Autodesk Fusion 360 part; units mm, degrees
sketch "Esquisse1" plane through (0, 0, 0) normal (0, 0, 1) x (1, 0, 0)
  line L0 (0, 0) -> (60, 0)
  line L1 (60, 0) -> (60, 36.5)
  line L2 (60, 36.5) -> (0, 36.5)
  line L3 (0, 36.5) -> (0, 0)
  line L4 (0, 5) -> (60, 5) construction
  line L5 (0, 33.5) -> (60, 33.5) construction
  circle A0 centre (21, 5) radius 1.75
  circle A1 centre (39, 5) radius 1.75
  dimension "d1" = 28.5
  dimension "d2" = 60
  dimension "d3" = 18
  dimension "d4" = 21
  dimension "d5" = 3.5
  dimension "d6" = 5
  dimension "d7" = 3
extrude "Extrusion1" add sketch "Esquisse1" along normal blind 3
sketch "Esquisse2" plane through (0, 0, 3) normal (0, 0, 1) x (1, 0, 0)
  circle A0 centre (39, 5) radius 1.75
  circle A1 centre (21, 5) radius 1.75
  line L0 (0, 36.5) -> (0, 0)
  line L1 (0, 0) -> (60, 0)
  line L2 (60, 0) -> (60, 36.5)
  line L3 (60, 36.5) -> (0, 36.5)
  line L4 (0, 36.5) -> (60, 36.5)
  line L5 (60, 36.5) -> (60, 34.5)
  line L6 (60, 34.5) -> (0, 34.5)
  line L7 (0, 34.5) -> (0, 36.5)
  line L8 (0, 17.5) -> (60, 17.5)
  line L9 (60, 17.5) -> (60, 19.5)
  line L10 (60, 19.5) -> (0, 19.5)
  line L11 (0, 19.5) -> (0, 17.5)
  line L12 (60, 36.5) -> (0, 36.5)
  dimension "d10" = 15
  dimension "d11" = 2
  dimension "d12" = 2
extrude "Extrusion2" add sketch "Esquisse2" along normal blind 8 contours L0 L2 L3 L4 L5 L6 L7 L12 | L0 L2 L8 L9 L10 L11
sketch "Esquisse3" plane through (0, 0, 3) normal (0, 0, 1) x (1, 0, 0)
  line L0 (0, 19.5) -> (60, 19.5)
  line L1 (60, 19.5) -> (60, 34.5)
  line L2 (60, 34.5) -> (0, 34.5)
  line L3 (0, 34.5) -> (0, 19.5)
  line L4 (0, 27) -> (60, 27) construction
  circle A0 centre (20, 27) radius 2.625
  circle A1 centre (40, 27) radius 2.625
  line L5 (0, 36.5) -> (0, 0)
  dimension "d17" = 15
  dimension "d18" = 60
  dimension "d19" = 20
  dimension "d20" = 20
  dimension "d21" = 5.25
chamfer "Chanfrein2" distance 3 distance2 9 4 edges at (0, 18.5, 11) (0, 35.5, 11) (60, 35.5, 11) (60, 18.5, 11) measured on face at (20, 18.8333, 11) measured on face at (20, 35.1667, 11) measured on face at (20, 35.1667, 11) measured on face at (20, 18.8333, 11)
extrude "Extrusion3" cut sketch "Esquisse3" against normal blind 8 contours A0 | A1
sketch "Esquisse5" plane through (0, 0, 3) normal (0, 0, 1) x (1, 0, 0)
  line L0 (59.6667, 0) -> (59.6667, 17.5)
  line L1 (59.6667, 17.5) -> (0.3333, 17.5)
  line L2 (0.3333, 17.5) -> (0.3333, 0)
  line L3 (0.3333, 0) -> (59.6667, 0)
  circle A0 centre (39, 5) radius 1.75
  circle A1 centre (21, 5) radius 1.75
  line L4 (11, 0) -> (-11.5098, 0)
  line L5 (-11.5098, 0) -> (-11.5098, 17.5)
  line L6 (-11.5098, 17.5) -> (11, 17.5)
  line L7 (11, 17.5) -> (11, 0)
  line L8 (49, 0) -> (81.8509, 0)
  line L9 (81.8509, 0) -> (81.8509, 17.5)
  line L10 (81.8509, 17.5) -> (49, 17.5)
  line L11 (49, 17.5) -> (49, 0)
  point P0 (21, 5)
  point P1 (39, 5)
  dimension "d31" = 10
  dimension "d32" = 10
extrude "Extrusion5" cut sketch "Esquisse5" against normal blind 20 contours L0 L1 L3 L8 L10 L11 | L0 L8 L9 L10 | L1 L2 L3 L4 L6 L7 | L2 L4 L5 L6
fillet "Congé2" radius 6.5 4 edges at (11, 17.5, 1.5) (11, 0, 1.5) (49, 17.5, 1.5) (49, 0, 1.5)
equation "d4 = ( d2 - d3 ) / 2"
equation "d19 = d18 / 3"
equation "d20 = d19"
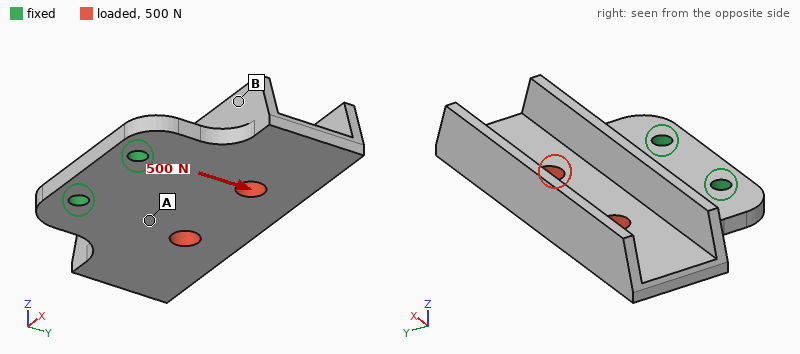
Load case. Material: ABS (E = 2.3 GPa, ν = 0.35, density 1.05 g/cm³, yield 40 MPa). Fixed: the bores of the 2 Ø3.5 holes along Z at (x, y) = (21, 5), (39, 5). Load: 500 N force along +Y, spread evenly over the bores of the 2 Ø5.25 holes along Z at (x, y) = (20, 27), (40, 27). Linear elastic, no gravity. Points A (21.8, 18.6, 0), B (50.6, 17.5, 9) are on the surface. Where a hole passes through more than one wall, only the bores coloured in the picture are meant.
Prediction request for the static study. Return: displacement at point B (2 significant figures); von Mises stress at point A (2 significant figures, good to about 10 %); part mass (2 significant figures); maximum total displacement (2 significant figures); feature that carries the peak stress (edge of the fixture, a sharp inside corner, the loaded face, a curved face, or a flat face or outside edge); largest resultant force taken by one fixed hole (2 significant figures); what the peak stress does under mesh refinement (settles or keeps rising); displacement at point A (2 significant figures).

36 µm
5.7 MPa
7.4 g
70 µm
edge of the fixture
250 N
keeps rising
37 µm
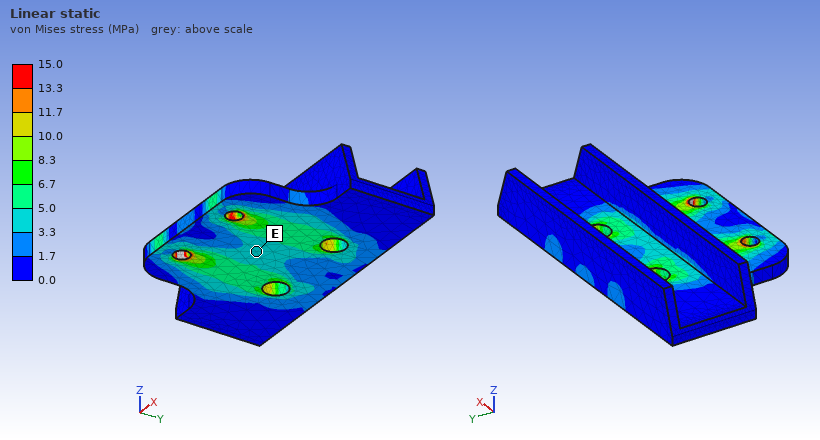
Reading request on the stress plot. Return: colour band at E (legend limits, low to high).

3.3 to 5.0 MPa
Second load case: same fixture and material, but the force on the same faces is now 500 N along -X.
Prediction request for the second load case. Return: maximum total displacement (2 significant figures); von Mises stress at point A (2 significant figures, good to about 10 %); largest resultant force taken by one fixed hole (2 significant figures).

0.51 mm
11 MPa
580 N
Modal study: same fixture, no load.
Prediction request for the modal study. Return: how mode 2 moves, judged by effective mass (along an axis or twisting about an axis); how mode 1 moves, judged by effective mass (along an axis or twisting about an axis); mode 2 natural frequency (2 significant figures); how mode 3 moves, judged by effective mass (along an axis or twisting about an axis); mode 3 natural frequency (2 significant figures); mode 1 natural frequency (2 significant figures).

twisting about Y
along Z
690 Hz
along X
2300 Hz
460 Hz
